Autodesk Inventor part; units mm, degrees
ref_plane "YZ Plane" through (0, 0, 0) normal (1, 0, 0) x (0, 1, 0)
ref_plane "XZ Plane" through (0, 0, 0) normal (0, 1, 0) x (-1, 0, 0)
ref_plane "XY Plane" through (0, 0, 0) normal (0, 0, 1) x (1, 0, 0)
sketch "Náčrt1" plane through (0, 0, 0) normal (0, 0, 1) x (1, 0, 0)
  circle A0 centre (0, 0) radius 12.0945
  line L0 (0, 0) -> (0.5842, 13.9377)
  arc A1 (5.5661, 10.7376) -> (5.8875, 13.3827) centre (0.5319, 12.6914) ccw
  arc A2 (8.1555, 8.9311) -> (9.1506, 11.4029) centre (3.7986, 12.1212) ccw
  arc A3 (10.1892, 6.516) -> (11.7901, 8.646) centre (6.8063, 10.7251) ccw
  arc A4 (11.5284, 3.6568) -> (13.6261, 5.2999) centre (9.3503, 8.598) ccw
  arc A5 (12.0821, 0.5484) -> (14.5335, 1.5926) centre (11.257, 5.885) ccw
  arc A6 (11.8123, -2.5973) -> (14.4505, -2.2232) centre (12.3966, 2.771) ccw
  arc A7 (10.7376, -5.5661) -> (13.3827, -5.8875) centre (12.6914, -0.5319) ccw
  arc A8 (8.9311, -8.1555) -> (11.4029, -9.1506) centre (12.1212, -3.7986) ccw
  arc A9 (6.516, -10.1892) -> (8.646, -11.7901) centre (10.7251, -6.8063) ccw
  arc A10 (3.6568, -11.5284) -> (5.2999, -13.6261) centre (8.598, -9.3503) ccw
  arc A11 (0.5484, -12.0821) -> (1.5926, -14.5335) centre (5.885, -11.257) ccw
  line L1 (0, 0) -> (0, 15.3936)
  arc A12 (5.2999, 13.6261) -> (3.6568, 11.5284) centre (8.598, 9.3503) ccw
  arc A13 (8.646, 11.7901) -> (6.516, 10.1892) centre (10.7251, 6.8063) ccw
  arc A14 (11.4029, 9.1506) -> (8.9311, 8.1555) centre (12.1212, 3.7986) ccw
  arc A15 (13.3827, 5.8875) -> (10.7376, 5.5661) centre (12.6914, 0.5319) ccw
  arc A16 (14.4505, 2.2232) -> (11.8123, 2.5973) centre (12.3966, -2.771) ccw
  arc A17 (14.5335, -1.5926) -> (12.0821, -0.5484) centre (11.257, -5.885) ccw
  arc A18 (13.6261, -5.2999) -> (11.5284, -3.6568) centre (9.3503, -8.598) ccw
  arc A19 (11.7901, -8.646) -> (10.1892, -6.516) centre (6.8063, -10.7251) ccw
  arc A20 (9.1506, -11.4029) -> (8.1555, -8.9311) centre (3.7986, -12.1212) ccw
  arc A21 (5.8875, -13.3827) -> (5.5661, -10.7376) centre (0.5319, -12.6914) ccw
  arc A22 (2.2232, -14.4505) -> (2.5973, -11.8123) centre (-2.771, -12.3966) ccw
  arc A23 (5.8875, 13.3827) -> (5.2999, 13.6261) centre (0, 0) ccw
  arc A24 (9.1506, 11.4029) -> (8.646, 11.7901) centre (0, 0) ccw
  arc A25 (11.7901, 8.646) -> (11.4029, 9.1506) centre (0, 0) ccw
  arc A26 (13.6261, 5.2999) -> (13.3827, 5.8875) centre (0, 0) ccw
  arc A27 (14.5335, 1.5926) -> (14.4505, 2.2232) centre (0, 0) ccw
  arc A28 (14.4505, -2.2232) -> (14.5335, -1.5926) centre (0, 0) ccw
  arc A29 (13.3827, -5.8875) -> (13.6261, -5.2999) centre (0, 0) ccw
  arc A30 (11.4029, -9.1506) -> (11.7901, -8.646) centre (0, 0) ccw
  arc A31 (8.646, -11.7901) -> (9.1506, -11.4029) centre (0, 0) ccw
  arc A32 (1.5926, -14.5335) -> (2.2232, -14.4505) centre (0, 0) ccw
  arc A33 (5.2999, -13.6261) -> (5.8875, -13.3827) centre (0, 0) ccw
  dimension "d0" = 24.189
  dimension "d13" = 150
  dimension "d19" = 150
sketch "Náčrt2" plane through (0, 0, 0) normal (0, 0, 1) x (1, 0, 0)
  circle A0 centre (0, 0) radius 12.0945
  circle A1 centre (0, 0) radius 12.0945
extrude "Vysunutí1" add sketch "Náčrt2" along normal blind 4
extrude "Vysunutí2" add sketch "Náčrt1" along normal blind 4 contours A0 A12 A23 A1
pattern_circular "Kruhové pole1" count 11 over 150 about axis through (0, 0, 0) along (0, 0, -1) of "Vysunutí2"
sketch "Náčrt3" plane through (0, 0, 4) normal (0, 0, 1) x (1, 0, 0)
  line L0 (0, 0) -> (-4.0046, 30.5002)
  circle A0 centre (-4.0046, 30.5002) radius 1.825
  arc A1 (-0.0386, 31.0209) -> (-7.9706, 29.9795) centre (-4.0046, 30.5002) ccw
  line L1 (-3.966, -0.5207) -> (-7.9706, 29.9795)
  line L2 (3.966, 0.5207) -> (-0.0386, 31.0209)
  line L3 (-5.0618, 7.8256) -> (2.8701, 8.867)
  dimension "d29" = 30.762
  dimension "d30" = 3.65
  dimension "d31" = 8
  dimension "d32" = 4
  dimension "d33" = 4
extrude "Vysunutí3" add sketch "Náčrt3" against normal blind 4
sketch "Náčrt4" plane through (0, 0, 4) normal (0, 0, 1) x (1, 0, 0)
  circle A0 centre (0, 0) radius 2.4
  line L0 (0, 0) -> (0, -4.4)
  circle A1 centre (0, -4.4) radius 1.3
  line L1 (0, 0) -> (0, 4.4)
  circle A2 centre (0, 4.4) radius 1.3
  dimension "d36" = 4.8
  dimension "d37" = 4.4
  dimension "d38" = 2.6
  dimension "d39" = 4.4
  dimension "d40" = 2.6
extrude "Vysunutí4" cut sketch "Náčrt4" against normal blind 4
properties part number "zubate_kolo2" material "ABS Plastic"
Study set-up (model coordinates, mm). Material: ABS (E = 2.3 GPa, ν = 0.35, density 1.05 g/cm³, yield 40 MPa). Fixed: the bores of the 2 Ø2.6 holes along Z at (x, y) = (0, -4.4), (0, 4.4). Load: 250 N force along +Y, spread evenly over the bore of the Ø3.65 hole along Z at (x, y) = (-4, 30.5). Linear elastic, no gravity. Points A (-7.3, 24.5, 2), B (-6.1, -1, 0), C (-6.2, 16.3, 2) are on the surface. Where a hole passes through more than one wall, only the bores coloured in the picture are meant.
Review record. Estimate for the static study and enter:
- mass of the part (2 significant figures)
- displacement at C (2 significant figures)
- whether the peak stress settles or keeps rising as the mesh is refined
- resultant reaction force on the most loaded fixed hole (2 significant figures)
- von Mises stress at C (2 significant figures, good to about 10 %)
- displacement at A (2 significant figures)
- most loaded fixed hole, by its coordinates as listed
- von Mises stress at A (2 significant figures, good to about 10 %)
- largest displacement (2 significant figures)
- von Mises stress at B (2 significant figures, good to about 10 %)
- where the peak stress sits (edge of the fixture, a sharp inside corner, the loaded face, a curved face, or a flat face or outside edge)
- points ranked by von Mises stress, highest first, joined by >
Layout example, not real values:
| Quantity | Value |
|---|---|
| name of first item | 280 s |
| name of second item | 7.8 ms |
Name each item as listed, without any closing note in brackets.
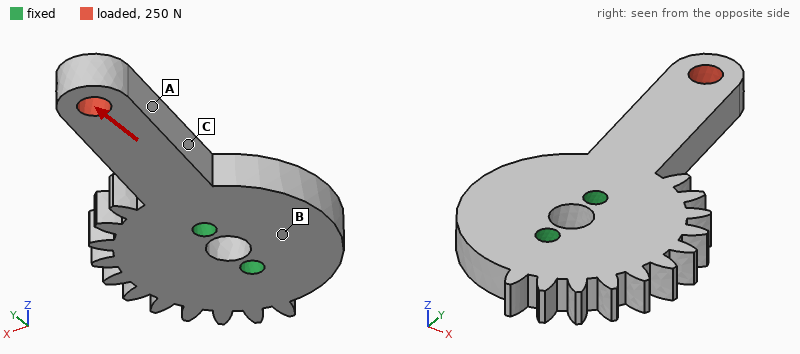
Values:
| Quantity | Value |
|---|---|
| mass of the part | 2.7 g |
| displacement at C | 0.15 mm |
| whether the peak stress settles or keeps rising as the mesh is refined | keeps rising |
| resultant reaction force on the most loaded fixed hole | 210 N |
| von Mises stress at C | 18 MPa |
| displacement at A | 0.31 mm |
| most loaded fixed hole, by its coordinates as listed | (0, 4.4) |
| von Mises stress at A | 13 MPa |
| largest displacement | 0.51 mm |
| von Mises stress at B | 3.5 MPa |
| where the peak stress sits | edge of the fixture |
| points ranked by von Mises stress, highest first, joined by > | C > A > B |
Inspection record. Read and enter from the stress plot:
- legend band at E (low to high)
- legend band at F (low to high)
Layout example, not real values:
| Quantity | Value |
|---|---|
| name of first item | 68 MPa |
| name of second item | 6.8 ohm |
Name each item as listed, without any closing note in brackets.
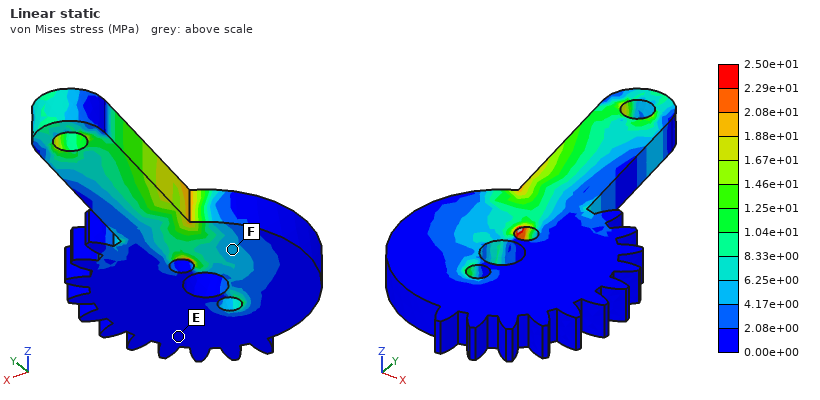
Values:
| Quantity | Value |
|---|---|
| legend band at E | 0.00e+00 to 2.08e+00 MPa |
| legend band at F | 4.17e+00 to 6.25e+00 MPa |
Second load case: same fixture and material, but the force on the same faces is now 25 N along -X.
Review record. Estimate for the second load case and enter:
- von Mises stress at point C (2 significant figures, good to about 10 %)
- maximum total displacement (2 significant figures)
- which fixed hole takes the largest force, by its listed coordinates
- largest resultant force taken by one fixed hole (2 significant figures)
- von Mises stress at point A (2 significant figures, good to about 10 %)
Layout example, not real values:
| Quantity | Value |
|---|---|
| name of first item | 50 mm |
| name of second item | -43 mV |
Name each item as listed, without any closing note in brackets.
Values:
| Quantity | Value |
|---|---|
| von Mises stress at point C | 7.9 MPa |
| maximum total displacement | 0.37 mm |
| which fixed hole takes the largest force, by its listed coordinates | (0, 4.4) |
| largest resultant force taken by one fixed hole | 73 N |
| von Mises stress at point A | 3.2 MPa |
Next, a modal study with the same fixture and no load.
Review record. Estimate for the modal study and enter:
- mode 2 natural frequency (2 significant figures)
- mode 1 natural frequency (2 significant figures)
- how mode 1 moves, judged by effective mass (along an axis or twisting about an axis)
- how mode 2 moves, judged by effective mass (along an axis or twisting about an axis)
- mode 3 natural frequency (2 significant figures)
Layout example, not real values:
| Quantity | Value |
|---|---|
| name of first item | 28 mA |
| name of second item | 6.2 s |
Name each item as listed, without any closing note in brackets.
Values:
| Quantity | Value |
|---|---|
| mode 2 natural frequency | 2700 Hz |
| mode 1 natural frequency | 1300 Hz |
| how mode 1 moves, judged by effective mass | along Z |
| how mode 2 moves, judged by effective mass | along X |
| mode 3 natural frequency | 5500 Hz |
